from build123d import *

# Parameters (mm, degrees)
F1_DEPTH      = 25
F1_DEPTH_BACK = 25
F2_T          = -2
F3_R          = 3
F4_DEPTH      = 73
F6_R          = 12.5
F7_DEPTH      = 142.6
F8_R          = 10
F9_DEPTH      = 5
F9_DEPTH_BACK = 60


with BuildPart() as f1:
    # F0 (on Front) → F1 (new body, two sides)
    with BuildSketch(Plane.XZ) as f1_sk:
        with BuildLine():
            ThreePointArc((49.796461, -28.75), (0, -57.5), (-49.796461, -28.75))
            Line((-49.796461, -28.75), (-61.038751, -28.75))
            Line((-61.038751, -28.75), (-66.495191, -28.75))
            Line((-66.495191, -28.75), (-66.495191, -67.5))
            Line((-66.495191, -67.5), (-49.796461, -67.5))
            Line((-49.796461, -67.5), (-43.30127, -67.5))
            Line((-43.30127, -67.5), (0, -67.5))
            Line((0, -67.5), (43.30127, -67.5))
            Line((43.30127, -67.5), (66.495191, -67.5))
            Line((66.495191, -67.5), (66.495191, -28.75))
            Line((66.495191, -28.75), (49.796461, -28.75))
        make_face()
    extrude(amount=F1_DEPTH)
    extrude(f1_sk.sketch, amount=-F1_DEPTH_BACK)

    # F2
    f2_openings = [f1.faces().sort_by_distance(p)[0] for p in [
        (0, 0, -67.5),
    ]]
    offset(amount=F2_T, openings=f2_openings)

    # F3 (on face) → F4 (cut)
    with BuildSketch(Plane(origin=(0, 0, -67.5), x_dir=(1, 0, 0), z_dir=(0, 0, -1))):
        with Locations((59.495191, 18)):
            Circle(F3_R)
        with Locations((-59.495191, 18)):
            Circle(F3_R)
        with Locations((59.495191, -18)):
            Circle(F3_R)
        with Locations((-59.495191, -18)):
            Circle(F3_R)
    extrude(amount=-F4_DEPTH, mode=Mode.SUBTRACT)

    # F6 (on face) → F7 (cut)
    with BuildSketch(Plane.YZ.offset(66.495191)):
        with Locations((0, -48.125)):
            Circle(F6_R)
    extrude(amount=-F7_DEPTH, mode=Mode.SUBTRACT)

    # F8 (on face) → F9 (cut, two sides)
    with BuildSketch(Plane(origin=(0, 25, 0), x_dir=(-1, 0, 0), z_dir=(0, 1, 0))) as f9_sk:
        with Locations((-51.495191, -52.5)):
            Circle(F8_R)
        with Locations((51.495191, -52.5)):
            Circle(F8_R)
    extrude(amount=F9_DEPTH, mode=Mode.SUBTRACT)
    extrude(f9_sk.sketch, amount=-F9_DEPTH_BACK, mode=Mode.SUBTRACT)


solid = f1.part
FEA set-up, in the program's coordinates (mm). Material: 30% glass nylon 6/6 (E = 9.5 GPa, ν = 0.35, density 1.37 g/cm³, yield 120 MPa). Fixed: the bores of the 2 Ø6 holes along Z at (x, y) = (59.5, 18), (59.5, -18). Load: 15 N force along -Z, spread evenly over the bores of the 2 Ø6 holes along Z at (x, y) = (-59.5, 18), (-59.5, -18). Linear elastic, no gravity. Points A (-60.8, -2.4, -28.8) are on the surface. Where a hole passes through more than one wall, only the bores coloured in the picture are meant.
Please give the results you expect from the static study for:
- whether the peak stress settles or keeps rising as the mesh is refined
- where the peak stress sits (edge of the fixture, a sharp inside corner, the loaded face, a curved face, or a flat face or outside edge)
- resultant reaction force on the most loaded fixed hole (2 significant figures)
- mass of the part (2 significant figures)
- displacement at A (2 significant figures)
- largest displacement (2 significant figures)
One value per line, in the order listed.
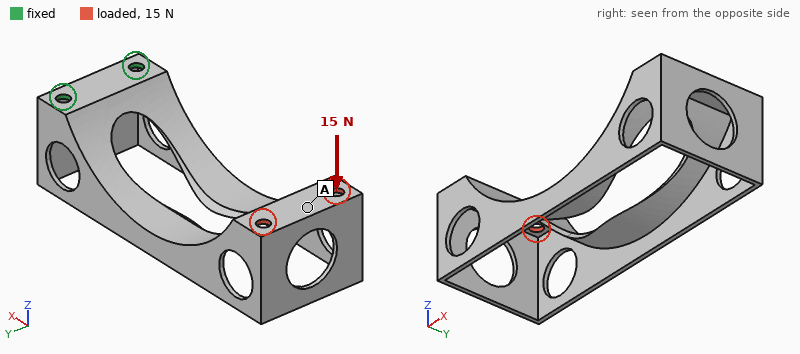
keeps rising
edge of the fixture
9.4 N
34 g
1.3 mm
1.4 mm
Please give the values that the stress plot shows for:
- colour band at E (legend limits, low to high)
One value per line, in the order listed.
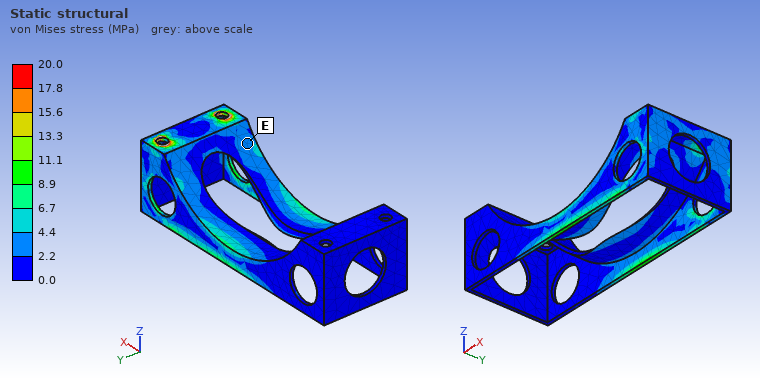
2.2 to 4.4 MPa
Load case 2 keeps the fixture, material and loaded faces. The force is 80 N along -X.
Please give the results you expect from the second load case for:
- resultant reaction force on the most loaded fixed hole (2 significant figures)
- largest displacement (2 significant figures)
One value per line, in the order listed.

40 N
1.7 mm
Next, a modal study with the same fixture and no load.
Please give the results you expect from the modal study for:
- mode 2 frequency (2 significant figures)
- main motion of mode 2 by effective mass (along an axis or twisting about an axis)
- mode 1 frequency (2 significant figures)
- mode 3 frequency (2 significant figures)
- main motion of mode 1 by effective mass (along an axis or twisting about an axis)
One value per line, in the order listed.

190 Hz
along Y
150 Hz
280 Hz
along Z
